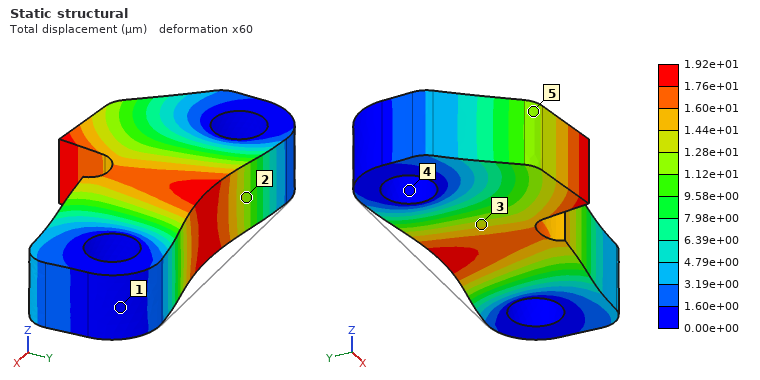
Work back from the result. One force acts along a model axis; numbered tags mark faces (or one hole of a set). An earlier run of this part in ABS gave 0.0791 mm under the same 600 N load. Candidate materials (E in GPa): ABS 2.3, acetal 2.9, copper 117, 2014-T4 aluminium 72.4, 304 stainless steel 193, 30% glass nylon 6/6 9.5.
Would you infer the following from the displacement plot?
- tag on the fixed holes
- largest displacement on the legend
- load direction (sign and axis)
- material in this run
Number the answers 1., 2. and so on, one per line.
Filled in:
1. 4
2. 1.92e+01 µm
3. -Y
4. 30% glass nylon 6/6
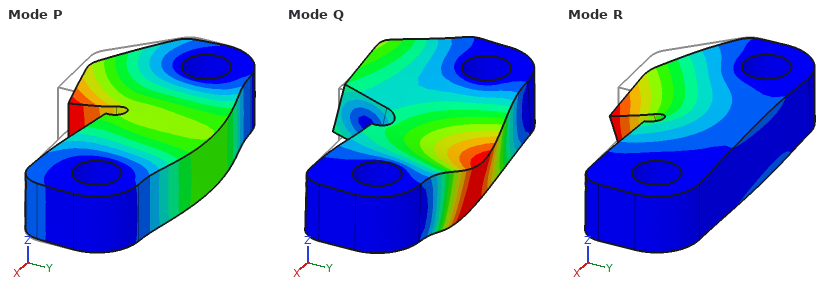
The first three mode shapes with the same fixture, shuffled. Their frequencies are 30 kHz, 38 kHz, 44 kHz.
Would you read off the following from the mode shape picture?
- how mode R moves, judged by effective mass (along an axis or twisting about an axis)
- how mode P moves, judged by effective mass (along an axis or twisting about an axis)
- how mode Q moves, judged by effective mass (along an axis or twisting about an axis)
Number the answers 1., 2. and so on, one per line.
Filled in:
1. along Z
2. along Y
3. along Z
